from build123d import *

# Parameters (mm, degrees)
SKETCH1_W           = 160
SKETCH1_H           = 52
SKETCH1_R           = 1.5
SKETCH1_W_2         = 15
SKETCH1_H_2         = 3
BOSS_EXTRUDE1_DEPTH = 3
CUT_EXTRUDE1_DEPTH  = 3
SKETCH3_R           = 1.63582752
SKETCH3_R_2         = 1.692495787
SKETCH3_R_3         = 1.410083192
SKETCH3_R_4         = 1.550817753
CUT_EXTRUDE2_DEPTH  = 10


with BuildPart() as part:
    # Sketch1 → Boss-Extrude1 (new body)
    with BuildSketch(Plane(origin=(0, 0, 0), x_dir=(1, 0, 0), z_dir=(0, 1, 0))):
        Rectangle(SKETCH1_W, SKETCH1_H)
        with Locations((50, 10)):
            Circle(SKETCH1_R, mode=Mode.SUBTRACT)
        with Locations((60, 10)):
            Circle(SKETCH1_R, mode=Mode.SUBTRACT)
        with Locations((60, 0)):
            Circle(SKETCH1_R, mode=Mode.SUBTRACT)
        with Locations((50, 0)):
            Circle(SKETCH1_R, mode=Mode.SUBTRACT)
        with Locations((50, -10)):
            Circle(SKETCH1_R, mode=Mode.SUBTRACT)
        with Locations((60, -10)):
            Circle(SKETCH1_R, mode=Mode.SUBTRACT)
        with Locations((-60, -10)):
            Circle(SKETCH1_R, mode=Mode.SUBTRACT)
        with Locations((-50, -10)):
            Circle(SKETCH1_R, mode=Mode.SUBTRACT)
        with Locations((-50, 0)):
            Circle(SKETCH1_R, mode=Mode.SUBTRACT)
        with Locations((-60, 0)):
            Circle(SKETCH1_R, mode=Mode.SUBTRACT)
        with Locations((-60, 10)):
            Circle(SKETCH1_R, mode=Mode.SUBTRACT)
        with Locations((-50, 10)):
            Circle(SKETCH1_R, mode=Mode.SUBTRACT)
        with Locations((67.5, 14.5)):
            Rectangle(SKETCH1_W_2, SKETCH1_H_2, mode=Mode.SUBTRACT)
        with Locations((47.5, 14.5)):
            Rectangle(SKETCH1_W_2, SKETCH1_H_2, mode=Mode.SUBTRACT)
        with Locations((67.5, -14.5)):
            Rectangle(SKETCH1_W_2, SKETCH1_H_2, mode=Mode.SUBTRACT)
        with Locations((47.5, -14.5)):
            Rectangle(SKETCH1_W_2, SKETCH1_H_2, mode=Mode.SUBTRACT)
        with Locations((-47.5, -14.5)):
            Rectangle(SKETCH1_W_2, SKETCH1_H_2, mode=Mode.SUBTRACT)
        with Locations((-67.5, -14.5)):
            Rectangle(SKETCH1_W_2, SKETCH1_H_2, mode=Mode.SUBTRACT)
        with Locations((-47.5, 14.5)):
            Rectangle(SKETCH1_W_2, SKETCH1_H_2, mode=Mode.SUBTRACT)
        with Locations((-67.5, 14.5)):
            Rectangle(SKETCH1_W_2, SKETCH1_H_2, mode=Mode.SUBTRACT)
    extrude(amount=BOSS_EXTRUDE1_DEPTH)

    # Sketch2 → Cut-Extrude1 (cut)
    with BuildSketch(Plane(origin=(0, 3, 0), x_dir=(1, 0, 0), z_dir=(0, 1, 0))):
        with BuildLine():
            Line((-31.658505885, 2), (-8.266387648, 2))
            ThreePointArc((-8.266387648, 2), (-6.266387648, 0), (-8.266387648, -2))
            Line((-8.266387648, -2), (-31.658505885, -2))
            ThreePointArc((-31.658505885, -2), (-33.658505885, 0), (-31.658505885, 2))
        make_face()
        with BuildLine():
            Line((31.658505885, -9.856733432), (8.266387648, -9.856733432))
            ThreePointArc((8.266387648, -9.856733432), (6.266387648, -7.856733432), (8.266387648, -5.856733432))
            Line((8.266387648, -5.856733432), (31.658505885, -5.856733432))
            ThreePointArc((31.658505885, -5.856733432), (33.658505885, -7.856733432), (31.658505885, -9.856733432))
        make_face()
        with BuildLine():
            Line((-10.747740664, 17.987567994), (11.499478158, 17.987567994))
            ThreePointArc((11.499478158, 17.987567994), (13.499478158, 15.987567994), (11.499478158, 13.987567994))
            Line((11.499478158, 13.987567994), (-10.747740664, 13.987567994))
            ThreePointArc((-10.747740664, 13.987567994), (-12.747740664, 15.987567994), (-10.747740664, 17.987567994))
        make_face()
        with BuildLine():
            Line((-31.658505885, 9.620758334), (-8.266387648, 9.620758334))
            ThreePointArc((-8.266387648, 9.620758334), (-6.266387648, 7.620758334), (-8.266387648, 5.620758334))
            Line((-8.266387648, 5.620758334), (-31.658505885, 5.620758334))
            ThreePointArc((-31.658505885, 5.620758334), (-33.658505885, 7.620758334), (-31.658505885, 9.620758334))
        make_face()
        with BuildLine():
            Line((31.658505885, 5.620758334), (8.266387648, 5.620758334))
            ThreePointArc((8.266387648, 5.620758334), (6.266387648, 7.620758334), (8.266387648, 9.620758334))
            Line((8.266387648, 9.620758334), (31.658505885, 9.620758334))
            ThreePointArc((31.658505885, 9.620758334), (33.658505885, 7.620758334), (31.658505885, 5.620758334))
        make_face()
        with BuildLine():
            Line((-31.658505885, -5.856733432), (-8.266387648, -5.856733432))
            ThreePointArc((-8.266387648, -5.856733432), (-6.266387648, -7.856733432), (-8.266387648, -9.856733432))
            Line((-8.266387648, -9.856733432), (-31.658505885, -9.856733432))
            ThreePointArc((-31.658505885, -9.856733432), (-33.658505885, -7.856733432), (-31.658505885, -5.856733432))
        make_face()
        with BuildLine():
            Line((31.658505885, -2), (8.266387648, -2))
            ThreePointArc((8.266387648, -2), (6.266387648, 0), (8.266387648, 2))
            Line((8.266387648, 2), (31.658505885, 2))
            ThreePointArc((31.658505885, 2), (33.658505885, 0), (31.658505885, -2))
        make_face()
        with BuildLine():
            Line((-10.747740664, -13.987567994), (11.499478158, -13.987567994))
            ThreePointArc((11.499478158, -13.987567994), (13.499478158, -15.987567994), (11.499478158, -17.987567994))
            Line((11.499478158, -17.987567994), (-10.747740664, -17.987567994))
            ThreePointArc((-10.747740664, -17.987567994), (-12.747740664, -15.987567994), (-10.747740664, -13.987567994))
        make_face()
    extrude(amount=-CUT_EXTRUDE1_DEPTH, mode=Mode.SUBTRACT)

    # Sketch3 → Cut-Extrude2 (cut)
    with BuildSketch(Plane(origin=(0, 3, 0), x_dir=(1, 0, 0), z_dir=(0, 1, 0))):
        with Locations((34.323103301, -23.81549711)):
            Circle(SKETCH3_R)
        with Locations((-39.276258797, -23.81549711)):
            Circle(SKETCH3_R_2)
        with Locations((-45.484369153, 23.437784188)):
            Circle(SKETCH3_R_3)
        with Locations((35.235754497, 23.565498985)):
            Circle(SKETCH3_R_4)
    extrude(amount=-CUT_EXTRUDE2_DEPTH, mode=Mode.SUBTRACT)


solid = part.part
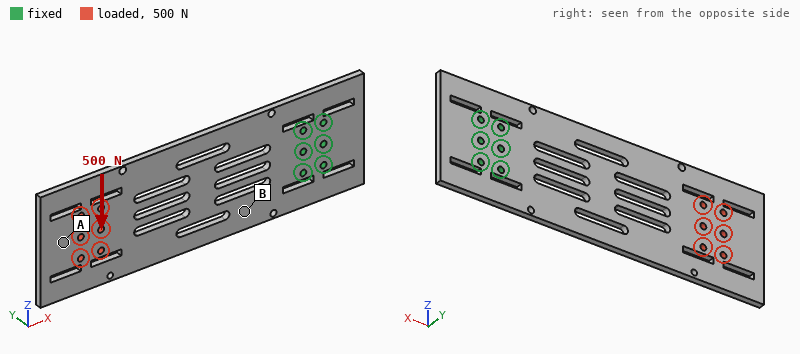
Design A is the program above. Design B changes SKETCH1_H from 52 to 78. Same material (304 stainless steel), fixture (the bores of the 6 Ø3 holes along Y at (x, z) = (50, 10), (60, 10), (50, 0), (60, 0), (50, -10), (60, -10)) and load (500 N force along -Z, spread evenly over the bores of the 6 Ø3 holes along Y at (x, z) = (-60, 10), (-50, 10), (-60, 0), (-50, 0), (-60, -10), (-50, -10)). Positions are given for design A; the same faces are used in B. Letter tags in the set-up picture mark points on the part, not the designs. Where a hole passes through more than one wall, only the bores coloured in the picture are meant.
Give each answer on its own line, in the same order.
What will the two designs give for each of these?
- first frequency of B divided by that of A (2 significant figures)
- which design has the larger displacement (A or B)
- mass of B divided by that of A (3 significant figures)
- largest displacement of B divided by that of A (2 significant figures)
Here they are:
0.98
A
1.59
0.56
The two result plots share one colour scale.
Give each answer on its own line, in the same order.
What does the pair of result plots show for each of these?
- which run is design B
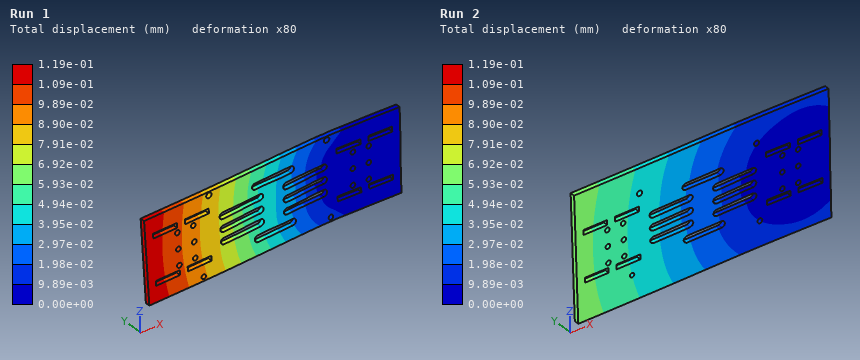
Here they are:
Run 2
